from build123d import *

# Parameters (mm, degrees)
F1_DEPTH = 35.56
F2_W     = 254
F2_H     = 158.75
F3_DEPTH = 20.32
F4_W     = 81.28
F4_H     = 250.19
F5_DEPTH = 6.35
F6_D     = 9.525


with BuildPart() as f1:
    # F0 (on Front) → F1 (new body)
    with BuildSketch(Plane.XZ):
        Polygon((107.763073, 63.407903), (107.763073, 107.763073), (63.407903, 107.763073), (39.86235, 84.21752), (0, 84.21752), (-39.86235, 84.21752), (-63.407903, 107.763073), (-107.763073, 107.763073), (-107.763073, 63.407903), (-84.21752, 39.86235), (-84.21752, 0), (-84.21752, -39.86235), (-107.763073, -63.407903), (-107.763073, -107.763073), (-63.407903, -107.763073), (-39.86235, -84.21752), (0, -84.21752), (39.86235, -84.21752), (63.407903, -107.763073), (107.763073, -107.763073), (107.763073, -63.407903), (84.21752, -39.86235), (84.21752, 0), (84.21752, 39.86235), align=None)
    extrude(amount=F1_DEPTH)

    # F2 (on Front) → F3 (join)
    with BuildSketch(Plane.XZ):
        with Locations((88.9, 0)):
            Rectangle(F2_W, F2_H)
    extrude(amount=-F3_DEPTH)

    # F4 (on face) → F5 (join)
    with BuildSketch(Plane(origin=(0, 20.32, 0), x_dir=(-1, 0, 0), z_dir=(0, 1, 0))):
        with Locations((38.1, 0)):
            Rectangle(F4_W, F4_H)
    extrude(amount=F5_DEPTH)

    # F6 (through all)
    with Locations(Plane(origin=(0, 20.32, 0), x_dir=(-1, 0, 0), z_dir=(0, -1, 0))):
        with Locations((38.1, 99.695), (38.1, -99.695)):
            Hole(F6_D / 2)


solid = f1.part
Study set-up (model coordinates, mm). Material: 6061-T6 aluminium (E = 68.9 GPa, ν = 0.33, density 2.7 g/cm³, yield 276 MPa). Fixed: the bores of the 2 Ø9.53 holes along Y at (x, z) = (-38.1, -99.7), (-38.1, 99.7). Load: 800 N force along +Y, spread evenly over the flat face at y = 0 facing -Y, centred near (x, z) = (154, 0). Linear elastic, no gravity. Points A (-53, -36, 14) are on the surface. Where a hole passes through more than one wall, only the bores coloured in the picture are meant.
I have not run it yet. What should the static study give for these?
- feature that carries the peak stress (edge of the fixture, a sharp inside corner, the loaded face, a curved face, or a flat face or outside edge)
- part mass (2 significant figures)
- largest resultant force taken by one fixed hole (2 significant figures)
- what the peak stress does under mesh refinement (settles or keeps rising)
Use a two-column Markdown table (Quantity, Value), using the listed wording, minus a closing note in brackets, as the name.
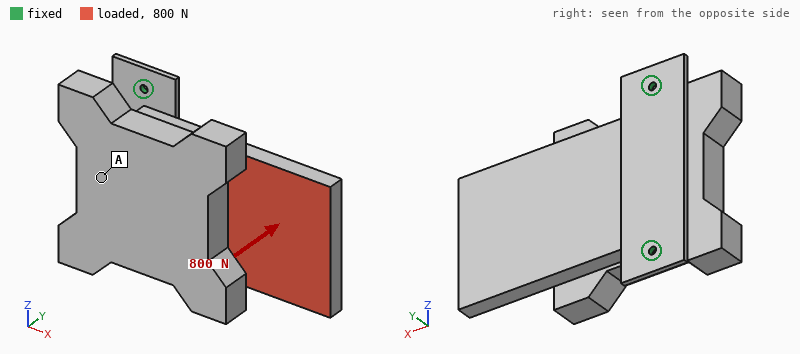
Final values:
| Quantity | Value |
|---|---|
| feature that carries the peak stress | edge of the fixture |
| part mass | 6.1 kg |
| largest resultant force taken by one fixed hole | 610 N |
| what the peak stress does under mesh refinement | keeps rising |
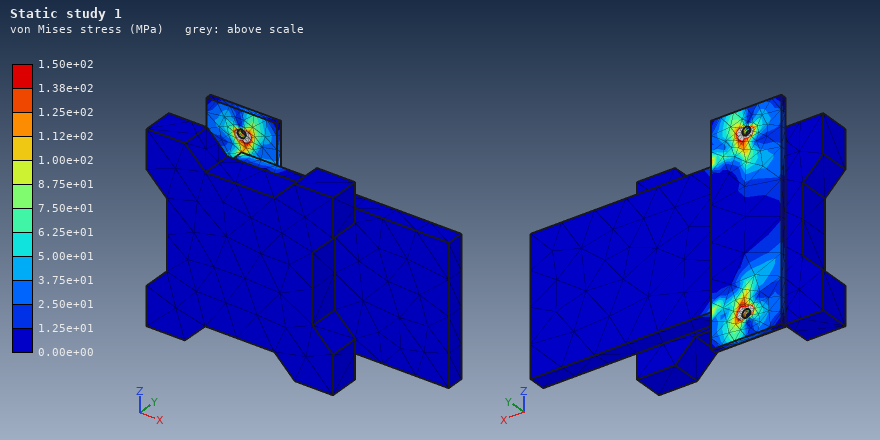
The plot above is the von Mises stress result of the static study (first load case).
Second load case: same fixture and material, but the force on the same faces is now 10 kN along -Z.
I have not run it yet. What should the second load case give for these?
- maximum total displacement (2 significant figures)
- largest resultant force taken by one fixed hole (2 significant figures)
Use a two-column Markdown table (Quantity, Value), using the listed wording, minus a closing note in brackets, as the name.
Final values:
| Quantity | Value |
|---|---|
| maximum total displacement | 0.19 mm |
| largest resultant force taken by one fixed hole | 11 kN |
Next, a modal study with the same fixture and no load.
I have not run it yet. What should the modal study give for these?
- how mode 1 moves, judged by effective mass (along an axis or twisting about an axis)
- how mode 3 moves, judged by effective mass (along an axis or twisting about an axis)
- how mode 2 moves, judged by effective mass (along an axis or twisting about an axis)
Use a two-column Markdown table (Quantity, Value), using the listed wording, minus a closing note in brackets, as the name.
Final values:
| Quantity | Value |
|---|---|
| how mode 1 moves, judged by effective mass | along Y |
| how mode 3 moves, judged by effective mass | along Z |
| how mode 2 moves, judged by effective mass | along Y |
